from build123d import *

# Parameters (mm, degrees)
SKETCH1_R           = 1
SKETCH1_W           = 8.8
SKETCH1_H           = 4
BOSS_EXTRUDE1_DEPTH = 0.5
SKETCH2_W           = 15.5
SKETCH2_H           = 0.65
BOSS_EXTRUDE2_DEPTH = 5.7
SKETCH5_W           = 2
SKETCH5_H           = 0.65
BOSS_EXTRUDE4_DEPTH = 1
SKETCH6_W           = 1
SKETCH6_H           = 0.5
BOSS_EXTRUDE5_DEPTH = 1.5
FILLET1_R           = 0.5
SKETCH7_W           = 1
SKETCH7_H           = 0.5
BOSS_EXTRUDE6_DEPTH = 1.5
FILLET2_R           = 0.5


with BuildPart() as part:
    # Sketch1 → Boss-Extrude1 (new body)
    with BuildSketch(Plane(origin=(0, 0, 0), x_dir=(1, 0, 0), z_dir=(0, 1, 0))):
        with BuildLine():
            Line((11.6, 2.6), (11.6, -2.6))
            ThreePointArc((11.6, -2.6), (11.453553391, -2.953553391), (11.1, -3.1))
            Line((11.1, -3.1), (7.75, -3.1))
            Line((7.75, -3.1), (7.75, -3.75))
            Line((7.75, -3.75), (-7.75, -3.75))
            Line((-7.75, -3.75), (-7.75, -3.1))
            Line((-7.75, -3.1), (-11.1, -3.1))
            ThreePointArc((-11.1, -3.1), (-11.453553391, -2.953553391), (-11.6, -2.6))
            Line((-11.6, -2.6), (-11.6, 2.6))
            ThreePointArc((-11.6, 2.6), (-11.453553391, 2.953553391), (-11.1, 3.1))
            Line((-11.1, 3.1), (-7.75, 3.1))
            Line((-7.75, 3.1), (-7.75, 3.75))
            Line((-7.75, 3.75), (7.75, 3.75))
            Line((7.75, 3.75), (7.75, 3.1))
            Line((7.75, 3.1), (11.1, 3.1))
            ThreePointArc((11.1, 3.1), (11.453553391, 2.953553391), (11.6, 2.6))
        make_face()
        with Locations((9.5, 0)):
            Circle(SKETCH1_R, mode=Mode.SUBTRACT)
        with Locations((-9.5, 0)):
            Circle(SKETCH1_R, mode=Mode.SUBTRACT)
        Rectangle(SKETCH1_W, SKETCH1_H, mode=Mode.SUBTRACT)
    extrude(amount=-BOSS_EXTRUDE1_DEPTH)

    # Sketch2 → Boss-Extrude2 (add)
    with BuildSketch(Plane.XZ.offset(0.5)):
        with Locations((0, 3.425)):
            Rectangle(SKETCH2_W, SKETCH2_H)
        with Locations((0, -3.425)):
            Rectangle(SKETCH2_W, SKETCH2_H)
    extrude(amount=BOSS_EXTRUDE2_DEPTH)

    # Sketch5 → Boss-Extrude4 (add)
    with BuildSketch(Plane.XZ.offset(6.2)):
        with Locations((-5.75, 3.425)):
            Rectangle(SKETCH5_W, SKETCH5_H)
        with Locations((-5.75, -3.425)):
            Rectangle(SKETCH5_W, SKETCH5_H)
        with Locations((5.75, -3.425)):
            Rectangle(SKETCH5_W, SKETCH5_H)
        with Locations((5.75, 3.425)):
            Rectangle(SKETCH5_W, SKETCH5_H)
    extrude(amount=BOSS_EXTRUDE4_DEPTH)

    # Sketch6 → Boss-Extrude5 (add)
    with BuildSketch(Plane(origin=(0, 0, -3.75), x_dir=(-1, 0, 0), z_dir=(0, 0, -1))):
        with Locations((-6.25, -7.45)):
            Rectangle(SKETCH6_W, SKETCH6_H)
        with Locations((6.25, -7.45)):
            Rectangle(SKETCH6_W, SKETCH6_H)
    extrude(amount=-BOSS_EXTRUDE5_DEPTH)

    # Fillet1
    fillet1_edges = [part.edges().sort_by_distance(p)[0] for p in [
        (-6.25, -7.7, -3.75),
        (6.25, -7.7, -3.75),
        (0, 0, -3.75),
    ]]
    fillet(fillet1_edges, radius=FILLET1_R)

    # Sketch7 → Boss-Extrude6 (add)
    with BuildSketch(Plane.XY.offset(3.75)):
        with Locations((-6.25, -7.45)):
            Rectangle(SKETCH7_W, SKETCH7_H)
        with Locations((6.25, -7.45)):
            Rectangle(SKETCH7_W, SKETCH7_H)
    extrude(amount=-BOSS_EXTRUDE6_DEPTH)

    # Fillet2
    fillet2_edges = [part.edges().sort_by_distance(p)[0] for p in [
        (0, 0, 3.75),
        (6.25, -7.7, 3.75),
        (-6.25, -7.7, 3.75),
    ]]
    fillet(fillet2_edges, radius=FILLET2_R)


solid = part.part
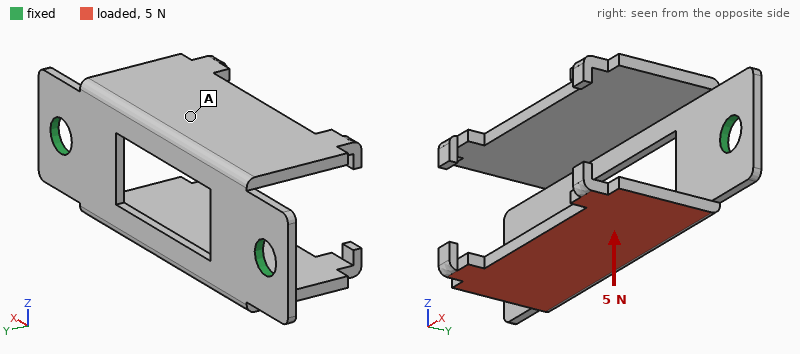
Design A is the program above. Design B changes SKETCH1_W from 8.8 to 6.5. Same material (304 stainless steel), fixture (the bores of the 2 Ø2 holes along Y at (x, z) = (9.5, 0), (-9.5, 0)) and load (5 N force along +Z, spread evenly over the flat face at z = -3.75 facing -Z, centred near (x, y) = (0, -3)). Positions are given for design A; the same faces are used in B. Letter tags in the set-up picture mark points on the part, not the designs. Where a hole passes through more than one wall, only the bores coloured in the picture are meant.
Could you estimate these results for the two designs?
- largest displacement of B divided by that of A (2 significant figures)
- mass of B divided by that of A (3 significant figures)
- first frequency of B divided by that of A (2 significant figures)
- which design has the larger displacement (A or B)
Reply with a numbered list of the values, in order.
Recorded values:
1. 0.84
2. 1.03
3. 1.1
4. A
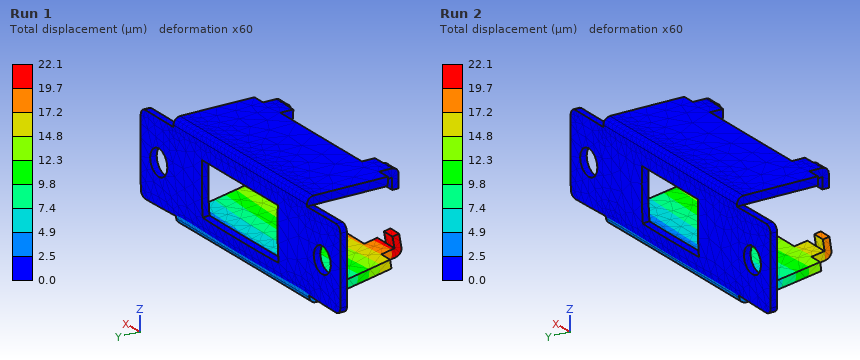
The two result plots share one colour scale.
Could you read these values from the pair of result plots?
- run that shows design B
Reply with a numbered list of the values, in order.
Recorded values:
1. Run 2
